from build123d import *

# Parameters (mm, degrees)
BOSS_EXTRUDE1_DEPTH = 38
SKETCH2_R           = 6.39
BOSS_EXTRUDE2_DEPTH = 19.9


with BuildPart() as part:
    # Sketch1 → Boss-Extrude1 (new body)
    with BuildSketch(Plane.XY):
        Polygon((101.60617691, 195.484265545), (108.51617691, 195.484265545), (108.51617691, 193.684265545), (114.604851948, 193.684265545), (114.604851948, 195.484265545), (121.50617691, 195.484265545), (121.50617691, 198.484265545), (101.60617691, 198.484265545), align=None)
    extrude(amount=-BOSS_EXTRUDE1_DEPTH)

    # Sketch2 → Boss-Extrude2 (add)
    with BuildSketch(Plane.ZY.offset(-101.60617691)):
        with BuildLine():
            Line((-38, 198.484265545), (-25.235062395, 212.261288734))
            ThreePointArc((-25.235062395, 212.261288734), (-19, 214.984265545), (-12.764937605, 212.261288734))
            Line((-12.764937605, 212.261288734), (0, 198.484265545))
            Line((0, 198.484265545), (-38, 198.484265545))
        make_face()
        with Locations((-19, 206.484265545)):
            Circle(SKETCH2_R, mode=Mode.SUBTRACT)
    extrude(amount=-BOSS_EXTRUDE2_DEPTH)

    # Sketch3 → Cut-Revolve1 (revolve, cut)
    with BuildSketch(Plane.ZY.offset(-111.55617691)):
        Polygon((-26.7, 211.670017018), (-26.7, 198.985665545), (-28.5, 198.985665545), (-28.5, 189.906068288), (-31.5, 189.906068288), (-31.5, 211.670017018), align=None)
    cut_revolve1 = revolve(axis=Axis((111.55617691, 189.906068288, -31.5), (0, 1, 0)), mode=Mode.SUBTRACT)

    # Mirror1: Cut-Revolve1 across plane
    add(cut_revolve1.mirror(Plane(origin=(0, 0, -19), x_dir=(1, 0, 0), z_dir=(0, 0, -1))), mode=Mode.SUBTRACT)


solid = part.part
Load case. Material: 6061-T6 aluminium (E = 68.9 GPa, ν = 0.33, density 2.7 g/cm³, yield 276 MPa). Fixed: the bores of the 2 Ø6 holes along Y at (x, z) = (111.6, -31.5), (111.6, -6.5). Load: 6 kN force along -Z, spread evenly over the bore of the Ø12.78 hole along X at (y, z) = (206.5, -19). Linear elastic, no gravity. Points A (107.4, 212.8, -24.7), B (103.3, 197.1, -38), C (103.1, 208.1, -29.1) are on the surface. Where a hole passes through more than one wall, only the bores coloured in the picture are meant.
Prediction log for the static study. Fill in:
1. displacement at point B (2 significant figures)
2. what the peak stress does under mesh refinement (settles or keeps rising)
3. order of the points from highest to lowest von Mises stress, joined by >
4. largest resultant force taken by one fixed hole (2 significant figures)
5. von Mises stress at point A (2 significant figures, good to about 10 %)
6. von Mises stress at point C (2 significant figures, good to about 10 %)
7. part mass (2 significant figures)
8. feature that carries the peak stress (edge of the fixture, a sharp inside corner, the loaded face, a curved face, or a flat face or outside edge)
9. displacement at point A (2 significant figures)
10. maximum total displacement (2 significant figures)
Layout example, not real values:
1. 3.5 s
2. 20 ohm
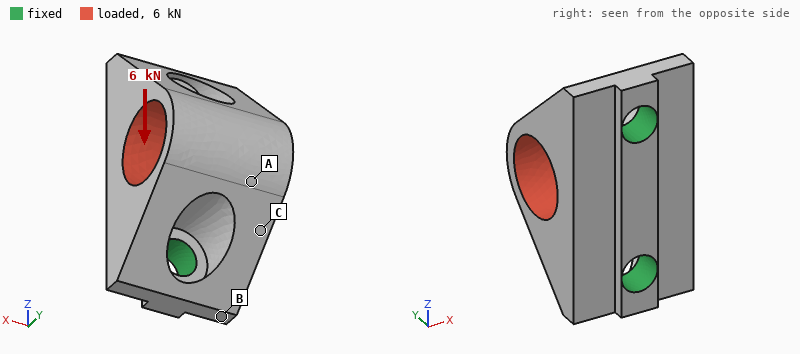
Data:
1. 14 µm
2. keeps rising
3. C > A > B
4. 3.6 kN
5. 63 MPa
6. 82 MPa
7. 17 g
8. edge of the fixture
9. 43 µm
10. 44 µm
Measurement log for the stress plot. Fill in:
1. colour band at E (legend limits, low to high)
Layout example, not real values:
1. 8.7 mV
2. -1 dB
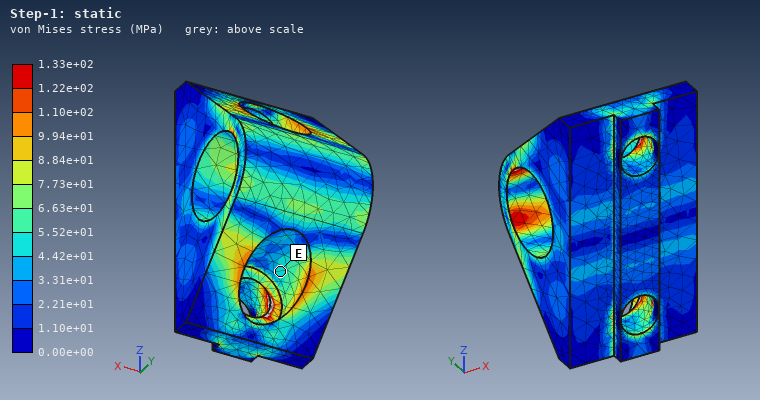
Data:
1. 4.42e+01 to 5.52e+01 MPa
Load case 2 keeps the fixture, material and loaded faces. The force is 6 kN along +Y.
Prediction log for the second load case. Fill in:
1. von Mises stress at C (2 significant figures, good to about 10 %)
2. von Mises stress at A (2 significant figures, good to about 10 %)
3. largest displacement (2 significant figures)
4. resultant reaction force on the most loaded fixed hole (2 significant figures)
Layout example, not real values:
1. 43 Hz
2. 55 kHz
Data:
1. 31 MPa
2. 21 MPa
3. 18 µm
4. 3.2 kN
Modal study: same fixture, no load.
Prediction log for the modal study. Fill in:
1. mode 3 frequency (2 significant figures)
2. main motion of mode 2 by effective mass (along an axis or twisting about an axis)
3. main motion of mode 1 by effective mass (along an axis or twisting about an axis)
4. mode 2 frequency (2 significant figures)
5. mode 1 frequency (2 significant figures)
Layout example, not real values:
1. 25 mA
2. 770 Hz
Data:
1. 30 kHz
2. along Z
3. along X
4. 26 kHz
5. 14 kHz
